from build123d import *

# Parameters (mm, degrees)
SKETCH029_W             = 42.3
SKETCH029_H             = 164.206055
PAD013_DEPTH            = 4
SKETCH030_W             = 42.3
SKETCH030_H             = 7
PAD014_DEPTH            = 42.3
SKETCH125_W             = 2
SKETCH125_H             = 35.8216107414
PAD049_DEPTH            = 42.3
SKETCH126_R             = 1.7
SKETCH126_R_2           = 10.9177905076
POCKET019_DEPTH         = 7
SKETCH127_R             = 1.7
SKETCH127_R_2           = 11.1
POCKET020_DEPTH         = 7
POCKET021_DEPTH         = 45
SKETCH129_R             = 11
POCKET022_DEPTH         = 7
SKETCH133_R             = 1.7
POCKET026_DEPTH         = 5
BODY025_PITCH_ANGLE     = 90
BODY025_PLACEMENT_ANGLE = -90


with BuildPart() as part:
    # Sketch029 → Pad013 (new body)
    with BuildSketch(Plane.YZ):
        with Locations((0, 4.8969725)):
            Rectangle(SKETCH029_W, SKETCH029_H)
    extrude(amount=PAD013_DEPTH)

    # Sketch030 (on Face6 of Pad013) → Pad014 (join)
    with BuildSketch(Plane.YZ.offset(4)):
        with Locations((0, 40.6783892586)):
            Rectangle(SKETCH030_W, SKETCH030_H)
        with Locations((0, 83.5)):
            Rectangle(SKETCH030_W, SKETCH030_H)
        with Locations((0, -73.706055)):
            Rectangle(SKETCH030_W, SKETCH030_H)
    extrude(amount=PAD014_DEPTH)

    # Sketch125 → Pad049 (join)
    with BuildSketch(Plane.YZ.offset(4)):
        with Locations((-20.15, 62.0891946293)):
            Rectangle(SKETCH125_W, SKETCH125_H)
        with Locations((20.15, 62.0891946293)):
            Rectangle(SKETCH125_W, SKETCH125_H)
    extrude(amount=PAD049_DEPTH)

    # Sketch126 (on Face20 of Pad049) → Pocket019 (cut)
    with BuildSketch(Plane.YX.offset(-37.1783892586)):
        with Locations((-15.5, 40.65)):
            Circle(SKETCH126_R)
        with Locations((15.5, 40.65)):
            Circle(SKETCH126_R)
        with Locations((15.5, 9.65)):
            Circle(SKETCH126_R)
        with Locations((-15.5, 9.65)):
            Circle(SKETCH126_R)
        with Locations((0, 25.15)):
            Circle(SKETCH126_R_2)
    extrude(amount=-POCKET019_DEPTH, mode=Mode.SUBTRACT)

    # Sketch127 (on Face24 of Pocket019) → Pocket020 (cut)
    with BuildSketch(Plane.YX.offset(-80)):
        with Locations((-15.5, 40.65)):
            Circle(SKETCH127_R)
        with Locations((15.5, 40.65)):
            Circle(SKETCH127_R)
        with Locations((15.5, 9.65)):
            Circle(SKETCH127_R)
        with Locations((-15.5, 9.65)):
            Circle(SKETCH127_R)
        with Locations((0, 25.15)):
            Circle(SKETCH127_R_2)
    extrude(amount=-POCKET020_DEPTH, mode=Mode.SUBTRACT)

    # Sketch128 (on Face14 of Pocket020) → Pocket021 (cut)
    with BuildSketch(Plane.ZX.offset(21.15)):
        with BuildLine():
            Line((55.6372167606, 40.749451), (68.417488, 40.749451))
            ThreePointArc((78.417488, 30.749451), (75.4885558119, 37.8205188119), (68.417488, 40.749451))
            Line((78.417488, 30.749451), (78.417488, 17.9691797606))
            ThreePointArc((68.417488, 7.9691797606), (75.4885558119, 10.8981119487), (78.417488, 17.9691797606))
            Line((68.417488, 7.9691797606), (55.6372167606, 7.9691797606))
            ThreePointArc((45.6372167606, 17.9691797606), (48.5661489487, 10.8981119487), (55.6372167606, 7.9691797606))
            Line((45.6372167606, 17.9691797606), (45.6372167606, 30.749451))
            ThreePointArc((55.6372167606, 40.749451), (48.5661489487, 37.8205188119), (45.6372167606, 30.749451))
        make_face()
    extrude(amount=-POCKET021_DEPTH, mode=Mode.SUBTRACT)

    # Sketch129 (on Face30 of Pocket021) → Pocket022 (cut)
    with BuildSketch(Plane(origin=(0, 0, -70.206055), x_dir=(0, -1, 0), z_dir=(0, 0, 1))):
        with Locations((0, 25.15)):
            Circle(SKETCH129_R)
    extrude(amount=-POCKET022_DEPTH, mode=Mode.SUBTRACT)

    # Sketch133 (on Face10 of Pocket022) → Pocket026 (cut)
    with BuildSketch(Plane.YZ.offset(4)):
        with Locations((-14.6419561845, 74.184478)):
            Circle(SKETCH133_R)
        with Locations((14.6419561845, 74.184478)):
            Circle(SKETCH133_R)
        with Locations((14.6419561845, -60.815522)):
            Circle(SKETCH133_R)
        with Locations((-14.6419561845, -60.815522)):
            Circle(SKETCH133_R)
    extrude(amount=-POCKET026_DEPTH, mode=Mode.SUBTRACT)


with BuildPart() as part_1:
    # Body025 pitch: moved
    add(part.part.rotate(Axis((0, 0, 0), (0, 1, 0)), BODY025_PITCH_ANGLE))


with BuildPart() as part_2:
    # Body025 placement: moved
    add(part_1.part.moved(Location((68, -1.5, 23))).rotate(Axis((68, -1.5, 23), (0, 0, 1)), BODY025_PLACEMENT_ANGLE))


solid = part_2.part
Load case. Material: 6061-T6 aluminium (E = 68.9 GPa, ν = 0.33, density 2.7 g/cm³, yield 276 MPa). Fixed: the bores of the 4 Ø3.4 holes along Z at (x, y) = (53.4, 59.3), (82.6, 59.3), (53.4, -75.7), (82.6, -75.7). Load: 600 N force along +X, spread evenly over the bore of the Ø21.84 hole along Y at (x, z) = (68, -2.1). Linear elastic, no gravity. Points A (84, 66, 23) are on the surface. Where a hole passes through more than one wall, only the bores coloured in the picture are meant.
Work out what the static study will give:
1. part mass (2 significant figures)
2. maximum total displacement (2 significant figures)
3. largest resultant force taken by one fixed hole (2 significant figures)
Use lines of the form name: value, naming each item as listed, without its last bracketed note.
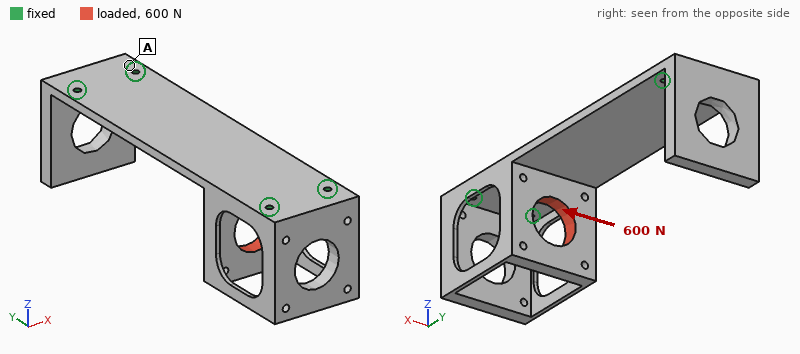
part mass: 160 g
maximum total displacement: 0.18 mm
largest resultant force taken by one fixed hole: 580 N
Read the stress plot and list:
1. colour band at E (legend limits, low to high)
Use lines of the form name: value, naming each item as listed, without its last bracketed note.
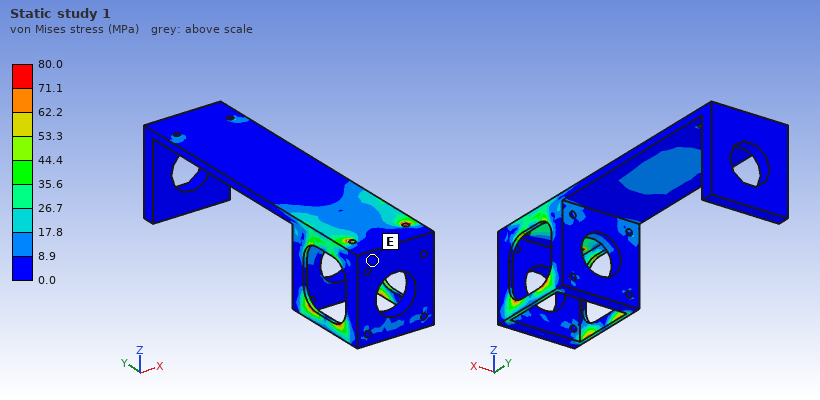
colour band at E: 0.0 to 8.9 MPa
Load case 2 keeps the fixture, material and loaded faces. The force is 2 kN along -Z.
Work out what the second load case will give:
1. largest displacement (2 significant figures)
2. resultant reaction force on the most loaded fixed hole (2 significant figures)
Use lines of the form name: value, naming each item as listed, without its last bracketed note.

largest displacement: 0.71 mm
resultant reaction force on the most loaded fixed hole: 900 N
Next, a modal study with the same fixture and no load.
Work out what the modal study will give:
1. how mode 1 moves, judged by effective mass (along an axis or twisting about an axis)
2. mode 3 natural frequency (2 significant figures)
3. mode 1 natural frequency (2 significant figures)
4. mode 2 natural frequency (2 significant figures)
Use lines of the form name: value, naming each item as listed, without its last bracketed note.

how mode 1 moves, judged by effective mass: along Z
mode 3 natural frequency: 1800 Hz
mode 1 natural frequency: 1000 Hz
mode 2 natural frequency: 1200 Hz
